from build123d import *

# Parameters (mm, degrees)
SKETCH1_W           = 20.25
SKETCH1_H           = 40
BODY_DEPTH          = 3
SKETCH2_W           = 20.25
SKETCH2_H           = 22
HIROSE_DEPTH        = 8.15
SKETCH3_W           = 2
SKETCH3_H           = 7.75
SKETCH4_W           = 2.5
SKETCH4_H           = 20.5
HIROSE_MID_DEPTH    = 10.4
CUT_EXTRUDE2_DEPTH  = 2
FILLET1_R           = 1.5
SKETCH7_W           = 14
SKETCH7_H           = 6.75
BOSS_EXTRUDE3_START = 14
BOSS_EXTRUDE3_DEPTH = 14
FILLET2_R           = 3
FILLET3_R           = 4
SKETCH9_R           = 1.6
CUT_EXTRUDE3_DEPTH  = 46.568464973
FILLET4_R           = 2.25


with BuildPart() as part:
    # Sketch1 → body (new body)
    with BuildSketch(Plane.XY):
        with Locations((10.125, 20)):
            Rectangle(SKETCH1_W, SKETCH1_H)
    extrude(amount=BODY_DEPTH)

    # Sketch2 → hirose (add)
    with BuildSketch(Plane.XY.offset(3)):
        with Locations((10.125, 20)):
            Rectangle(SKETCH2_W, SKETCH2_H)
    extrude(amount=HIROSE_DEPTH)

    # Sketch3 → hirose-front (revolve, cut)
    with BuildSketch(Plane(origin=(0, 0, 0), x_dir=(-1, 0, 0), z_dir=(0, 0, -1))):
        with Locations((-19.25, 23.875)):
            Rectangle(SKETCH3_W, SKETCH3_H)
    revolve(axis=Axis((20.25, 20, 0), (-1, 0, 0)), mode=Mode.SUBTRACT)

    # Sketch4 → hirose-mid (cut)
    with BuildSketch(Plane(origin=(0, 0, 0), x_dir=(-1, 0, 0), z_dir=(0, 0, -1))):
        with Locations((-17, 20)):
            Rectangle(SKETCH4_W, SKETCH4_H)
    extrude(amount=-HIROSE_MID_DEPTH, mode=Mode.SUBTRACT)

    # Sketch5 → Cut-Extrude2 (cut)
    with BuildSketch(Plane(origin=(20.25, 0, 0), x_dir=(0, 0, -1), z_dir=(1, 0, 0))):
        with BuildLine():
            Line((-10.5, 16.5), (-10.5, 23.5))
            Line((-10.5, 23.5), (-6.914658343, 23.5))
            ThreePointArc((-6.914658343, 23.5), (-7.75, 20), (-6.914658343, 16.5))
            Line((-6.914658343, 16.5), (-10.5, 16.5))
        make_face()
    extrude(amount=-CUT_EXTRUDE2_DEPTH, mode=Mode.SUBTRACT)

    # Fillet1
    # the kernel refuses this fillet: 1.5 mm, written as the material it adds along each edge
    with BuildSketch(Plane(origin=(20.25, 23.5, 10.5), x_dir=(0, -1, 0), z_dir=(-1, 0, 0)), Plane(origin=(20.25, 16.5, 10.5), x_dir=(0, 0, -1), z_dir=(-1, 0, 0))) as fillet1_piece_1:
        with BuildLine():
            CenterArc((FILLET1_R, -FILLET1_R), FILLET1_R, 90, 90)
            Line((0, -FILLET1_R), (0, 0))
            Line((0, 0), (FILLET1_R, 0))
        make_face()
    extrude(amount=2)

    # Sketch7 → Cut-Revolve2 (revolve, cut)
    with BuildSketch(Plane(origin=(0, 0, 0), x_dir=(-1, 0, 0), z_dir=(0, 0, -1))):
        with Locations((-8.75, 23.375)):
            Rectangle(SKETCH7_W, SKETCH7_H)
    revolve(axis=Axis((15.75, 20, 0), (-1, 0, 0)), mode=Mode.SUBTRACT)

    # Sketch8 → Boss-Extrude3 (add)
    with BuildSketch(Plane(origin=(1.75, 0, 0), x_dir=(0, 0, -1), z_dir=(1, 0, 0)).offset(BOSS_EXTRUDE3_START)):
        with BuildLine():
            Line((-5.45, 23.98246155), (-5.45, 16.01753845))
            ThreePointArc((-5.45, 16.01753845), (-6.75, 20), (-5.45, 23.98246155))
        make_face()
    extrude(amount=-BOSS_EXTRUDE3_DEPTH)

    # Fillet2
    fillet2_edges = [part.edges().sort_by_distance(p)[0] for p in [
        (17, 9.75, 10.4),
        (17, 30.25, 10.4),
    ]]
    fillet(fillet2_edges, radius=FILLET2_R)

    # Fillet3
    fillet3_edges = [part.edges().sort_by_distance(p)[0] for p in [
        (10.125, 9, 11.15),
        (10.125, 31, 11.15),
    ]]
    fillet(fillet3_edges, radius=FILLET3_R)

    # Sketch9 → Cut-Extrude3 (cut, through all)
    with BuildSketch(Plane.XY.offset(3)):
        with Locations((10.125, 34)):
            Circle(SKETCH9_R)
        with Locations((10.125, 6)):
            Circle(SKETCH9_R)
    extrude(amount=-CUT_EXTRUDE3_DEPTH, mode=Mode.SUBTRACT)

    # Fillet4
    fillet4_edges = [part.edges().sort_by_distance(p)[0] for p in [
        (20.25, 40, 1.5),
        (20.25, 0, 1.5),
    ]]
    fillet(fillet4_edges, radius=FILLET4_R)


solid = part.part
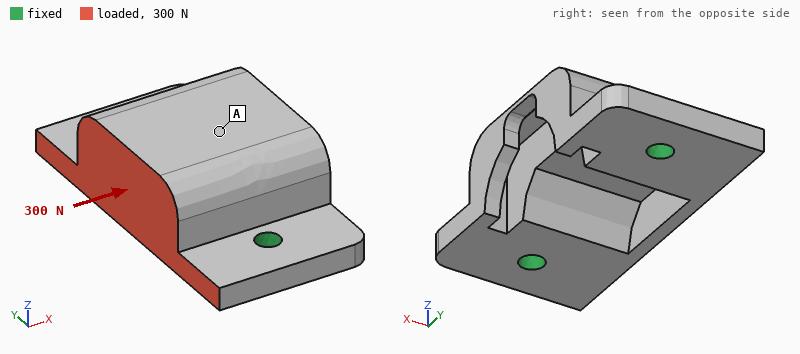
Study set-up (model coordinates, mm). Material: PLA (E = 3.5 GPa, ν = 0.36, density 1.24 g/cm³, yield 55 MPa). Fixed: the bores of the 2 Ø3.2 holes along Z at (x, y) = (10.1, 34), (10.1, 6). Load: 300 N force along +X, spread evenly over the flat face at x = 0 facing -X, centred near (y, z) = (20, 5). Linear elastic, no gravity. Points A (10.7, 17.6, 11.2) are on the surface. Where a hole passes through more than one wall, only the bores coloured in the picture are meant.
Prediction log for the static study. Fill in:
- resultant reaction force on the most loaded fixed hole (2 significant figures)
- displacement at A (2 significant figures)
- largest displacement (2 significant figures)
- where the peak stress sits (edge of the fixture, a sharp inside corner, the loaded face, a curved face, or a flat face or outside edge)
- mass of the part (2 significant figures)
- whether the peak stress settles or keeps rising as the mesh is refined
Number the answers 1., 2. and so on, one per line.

1. 160 N
2. 0.11 mm
3. 0.14 mm
4. edge of the fixture
5. 5.2 g
6. keeps rising
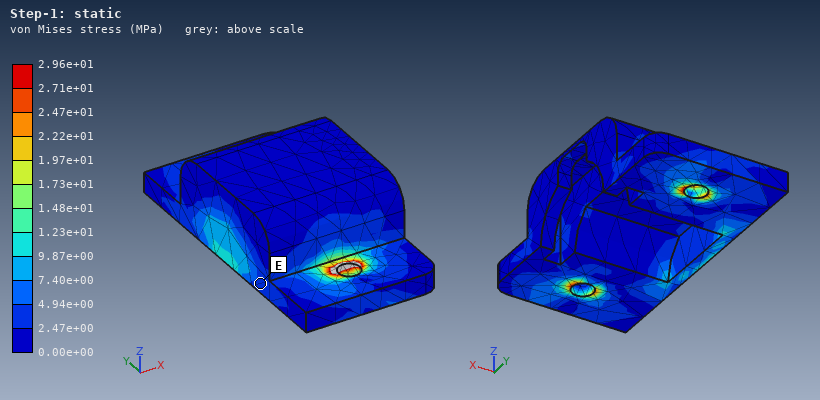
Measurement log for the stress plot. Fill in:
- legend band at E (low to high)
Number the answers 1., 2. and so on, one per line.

1. 2.47e+00 to 4.94e+00 MPa
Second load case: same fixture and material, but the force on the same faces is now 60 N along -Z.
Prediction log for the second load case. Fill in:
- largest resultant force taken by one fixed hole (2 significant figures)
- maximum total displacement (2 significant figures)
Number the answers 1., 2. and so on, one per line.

1. 34 N
2. 79 µm
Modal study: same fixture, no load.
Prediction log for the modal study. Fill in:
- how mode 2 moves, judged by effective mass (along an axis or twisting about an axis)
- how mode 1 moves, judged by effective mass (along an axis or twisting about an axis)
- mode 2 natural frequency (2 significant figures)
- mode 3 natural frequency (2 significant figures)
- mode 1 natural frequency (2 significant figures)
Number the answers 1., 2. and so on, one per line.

1. along Z
2. along X
3. 7800 Hz
4. 8300 Hz
5. 3100 Hz
